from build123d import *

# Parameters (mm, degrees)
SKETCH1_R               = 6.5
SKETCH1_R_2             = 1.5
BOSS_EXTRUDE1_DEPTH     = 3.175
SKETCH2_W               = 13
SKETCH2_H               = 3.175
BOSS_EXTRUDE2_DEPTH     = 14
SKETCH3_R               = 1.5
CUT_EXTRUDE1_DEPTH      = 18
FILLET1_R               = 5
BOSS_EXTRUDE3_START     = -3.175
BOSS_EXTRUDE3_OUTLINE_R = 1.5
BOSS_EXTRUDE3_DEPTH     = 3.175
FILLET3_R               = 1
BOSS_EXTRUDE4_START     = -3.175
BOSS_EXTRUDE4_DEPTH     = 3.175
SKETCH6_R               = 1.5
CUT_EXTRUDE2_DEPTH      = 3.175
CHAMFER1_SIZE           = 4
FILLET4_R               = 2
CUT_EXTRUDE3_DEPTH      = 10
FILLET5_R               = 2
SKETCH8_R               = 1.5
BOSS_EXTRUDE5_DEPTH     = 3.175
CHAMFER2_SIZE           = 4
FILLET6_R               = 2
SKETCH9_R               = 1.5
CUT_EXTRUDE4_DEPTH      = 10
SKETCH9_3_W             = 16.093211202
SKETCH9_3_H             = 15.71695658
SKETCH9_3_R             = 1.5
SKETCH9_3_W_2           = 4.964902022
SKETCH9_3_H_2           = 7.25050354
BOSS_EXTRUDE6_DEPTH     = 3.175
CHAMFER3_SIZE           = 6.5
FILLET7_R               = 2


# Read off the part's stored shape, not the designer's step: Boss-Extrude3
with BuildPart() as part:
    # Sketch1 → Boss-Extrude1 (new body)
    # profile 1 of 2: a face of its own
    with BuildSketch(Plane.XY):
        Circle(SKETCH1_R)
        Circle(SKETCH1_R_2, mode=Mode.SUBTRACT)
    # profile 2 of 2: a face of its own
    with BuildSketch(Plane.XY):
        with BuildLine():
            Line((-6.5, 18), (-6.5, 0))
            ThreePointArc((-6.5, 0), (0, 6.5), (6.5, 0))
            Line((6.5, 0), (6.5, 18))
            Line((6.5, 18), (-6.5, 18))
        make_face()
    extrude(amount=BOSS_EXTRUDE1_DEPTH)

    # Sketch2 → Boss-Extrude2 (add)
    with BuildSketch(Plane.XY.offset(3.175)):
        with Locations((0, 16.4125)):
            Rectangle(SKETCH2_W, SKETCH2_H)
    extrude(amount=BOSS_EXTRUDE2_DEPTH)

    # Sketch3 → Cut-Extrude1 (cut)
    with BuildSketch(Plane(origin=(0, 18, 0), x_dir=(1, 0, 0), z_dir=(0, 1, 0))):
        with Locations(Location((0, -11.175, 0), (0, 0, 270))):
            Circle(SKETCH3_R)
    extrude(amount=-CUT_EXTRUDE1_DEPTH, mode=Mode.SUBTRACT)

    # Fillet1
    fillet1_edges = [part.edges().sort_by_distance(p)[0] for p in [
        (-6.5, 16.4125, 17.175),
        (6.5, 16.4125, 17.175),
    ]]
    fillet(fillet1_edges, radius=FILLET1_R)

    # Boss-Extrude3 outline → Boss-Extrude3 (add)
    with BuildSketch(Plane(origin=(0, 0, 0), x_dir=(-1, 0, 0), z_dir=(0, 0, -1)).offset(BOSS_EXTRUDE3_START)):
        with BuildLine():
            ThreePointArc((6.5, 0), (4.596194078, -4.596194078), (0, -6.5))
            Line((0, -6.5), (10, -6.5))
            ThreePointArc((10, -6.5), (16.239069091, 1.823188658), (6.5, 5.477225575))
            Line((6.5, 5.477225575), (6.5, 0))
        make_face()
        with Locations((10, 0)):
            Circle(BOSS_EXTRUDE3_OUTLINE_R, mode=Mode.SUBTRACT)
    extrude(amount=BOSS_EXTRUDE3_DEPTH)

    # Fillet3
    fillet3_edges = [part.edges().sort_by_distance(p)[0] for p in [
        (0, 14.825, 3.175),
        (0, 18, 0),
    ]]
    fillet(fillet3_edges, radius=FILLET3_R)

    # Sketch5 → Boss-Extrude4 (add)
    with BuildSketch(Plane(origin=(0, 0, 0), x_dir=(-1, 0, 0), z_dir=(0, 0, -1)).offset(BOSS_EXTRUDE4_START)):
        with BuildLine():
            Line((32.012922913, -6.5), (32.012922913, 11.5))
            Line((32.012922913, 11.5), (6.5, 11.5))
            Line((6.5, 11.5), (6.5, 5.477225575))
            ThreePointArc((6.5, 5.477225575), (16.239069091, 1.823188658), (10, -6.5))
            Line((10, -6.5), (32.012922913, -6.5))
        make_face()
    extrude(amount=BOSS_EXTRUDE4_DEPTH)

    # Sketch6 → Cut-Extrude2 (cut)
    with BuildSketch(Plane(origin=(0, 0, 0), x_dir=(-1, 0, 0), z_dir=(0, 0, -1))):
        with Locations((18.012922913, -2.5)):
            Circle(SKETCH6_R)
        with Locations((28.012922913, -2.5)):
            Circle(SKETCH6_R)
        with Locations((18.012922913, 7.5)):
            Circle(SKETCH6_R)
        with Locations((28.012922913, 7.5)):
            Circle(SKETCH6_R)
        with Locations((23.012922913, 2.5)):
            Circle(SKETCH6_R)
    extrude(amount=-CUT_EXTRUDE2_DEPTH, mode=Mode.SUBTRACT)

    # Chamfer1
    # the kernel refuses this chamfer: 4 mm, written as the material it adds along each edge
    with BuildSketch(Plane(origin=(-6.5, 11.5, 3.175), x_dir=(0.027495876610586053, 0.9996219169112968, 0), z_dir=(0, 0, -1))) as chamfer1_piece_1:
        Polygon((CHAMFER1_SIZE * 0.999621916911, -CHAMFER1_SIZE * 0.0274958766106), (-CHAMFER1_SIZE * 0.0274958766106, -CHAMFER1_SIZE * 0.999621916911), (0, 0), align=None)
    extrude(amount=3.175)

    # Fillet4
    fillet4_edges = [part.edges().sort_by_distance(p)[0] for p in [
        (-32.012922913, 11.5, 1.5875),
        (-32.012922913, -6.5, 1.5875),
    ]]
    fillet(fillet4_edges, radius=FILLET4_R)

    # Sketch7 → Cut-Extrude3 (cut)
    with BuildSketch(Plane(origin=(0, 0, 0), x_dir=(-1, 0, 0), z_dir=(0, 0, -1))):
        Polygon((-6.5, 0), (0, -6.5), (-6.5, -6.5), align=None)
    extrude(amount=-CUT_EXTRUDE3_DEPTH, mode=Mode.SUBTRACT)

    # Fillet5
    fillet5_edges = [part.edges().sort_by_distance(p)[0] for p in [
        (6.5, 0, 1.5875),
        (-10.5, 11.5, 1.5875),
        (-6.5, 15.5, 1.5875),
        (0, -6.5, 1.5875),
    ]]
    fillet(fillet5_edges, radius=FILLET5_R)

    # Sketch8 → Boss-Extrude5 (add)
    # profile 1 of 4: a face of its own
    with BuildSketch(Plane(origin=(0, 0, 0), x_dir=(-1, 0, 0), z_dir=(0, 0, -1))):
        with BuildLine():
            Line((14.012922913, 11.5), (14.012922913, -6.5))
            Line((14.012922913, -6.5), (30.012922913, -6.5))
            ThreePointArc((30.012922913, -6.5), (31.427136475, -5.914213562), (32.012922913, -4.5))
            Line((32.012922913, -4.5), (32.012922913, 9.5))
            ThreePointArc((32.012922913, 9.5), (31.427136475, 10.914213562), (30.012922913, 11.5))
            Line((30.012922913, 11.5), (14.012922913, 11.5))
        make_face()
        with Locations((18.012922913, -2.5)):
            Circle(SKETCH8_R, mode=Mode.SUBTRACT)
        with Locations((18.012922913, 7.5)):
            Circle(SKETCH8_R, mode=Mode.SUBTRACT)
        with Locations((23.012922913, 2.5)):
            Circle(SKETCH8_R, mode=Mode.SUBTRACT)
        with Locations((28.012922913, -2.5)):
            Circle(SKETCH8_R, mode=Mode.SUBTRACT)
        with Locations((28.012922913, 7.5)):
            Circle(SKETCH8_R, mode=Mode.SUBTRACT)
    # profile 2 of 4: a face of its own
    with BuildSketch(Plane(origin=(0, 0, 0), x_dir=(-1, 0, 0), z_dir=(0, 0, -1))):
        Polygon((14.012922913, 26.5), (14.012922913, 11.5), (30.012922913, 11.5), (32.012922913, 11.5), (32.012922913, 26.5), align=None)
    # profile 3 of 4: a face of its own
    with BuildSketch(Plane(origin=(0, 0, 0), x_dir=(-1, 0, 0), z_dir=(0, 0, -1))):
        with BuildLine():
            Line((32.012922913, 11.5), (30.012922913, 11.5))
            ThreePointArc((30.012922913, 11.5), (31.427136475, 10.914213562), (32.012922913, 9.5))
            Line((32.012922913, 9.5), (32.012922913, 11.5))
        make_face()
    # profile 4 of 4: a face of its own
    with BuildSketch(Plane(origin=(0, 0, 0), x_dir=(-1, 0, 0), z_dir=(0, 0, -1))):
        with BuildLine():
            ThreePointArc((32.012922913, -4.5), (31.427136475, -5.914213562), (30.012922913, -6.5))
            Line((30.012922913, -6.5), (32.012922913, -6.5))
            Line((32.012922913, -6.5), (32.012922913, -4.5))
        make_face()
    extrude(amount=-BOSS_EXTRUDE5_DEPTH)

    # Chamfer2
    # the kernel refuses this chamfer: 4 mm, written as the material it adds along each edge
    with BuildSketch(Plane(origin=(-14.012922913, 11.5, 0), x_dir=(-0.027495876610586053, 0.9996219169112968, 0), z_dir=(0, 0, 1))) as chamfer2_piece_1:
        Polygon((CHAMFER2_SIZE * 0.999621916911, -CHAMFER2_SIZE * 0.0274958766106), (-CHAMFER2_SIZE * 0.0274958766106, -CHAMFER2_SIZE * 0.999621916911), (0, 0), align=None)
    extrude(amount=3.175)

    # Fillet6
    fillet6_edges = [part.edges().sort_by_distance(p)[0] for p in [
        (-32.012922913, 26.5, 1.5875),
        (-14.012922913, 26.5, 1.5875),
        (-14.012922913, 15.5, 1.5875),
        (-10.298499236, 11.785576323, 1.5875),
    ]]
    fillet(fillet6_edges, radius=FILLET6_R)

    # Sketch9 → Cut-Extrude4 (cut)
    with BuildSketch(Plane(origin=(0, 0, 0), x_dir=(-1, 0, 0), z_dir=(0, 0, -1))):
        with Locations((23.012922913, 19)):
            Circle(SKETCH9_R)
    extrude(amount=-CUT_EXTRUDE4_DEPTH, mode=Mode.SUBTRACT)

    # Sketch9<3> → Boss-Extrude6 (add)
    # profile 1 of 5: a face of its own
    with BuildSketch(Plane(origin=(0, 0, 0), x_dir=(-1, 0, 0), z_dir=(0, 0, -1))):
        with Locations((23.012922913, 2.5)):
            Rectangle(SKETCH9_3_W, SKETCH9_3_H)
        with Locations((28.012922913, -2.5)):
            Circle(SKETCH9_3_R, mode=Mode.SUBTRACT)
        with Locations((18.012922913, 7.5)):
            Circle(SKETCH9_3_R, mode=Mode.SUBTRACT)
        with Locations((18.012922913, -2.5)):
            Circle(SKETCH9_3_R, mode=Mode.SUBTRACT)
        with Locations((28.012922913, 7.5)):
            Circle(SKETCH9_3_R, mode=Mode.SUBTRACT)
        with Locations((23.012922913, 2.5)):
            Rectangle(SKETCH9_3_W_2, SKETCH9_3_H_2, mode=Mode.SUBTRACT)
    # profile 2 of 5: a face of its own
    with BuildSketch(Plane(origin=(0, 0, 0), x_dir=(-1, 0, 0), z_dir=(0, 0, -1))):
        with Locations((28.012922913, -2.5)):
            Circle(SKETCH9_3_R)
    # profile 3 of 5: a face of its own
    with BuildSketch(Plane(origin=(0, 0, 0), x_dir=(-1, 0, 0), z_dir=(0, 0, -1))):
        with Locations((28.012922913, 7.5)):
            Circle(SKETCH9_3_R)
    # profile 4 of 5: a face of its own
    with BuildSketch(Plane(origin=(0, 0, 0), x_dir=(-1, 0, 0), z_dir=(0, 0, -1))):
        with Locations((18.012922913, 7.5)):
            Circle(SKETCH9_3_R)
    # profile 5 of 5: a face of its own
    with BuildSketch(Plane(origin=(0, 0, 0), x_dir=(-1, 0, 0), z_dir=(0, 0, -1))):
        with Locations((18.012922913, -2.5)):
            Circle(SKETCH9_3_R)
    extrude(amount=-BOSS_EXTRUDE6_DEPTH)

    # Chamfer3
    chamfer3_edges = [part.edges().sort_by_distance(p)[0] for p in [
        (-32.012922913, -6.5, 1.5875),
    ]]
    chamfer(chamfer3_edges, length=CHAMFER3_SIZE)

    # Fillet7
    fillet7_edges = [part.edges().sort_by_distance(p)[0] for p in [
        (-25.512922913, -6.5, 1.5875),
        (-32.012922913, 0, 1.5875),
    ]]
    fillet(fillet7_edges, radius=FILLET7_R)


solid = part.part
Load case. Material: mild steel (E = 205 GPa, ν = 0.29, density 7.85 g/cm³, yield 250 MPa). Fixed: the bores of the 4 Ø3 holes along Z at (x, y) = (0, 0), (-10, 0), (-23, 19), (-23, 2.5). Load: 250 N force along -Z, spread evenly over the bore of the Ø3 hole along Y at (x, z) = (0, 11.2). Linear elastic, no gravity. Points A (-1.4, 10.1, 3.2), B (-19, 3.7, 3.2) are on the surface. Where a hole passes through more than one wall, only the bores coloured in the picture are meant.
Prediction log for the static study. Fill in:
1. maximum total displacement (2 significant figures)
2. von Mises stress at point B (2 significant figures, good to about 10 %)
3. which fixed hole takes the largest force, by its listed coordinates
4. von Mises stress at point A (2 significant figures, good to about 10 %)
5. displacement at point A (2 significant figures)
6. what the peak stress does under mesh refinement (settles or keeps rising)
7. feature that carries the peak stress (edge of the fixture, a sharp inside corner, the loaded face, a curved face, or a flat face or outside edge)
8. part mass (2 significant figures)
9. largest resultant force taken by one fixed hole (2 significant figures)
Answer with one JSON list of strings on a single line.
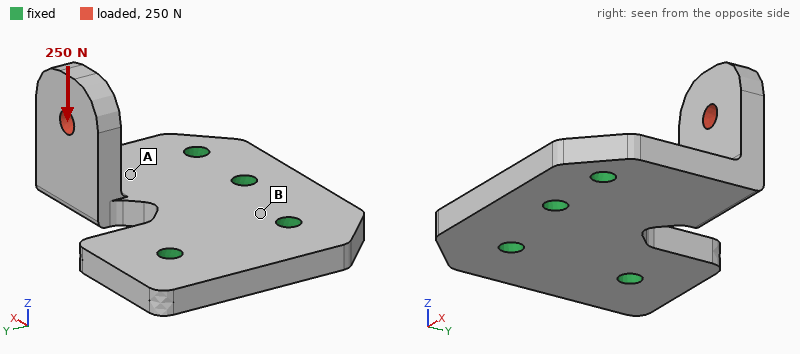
["56 µm", "12 MPa", "(0, 0)", "53 MPa", "12 µm", "keeps rising", "edge of the fixture", "29 g", "200 N"]
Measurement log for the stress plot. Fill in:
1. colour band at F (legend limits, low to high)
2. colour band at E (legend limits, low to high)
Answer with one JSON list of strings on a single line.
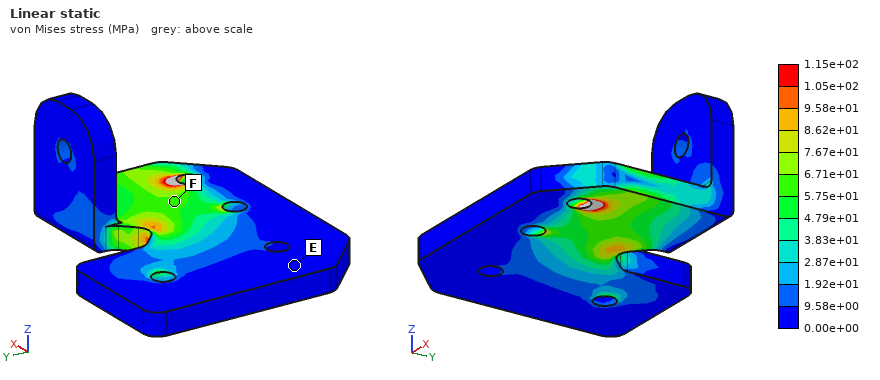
["5.75e+01 to 6.71e+01 MPa", "0.00e+00 to 9.58e+00 MPa"]
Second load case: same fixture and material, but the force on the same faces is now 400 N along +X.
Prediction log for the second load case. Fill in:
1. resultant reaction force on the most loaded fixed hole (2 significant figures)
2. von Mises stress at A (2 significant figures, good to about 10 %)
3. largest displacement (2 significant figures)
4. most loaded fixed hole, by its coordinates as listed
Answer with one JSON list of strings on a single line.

["390 N", "100 MPa", "55 µm", "(0, 0)"]
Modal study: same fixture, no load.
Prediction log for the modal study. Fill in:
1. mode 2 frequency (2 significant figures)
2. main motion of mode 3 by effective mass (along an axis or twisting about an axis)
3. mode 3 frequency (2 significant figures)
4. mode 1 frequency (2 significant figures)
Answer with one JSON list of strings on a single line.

["8700 Hz", "along Z", "13 kHz", "4700 Hz"]
